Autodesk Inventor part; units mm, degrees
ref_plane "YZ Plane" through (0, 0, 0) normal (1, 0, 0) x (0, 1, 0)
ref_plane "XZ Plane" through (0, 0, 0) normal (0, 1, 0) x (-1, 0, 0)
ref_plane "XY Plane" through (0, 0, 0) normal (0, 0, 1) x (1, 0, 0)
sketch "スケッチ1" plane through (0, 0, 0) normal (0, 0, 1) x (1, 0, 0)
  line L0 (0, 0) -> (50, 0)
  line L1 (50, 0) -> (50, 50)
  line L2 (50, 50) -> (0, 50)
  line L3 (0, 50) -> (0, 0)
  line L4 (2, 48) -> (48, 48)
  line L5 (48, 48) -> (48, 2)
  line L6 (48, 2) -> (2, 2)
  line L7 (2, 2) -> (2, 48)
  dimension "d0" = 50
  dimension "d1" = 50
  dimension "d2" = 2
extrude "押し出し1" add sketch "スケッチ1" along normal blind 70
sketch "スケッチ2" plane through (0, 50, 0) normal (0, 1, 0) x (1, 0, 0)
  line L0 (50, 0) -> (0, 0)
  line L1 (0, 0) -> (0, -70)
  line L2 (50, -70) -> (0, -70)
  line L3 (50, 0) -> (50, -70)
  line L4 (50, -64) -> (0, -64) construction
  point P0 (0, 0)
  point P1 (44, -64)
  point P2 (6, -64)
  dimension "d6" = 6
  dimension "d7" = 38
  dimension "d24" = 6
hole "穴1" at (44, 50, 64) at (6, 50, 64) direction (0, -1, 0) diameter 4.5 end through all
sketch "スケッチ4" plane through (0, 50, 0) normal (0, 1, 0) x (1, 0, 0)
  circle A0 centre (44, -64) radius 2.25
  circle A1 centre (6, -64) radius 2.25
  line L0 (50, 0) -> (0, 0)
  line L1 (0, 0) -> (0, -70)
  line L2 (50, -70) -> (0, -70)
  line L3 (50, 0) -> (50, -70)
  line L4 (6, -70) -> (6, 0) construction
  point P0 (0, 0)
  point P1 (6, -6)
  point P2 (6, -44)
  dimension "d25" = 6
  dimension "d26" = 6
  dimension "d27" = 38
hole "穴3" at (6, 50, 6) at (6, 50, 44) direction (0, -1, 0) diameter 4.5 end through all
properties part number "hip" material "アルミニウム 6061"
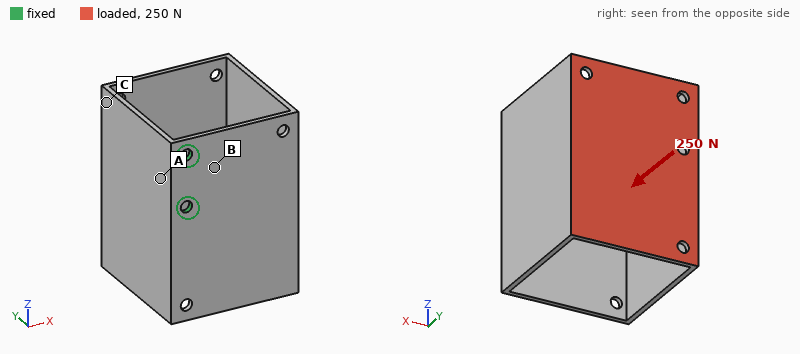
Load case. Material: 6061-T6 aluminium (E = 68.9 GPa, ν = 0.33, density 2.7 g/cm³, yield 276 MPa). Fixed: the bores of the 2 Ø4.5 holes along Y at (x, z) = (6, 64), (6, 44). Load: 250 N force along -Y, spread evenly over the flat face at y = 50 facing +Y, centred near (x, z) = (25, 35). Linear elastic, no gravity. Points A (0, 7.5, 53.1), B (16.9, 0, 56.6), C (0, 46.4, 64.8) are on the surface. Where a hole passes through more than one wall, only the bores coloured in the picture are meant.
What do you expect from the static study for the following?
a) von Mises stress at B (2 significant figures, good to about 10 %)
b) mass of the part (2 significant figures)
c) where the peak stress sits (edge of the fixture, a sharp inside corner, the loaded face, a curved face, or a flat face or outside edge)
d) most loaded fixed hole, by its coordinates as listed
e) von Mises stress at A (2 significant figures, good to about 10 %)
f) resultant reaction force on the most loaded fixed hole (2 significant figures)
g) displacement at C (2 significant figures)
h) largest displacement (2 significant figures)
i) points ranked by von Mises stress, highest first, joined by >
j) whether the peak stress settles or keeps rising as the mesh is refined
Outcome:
74 MPa
72 g
edge of the fixture
(6, 44)
45 MPa
310 N
0.71 mm
1.1 mm
B > A > C
keeps rising
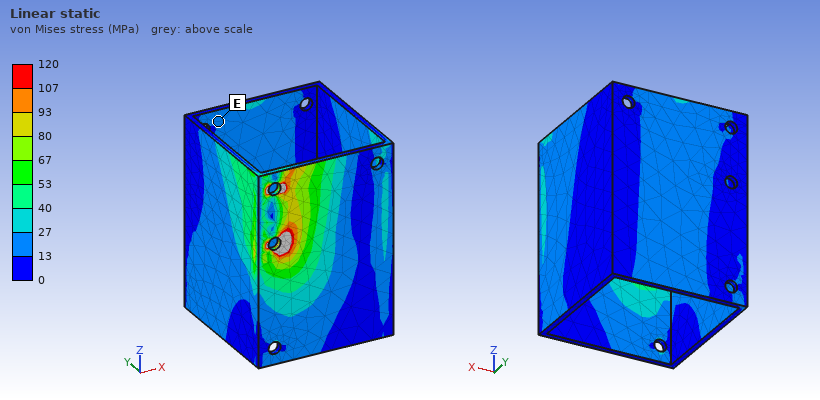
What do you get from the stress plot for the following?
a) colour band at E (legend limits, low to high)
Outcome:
13 to 27 MPa
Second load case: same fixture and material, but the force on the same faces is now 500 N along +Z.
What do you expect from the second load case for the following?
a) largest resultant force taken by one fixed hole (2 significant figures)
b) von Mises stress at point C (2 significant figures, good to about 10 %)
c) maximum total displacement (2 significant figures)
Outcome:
1.2 kN
44 MPa
1.0 mm
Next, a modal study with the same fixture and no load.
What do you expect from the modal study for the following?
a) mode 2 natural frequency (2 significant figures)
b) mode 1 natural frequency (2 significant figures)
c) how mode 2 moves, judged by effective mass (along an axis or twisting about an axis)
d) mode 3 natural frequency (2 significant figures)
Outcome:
660 Hz
260 Hz
along Z
800 Hz
